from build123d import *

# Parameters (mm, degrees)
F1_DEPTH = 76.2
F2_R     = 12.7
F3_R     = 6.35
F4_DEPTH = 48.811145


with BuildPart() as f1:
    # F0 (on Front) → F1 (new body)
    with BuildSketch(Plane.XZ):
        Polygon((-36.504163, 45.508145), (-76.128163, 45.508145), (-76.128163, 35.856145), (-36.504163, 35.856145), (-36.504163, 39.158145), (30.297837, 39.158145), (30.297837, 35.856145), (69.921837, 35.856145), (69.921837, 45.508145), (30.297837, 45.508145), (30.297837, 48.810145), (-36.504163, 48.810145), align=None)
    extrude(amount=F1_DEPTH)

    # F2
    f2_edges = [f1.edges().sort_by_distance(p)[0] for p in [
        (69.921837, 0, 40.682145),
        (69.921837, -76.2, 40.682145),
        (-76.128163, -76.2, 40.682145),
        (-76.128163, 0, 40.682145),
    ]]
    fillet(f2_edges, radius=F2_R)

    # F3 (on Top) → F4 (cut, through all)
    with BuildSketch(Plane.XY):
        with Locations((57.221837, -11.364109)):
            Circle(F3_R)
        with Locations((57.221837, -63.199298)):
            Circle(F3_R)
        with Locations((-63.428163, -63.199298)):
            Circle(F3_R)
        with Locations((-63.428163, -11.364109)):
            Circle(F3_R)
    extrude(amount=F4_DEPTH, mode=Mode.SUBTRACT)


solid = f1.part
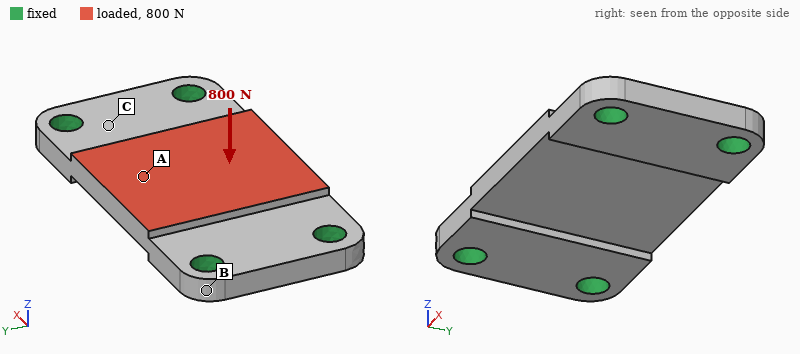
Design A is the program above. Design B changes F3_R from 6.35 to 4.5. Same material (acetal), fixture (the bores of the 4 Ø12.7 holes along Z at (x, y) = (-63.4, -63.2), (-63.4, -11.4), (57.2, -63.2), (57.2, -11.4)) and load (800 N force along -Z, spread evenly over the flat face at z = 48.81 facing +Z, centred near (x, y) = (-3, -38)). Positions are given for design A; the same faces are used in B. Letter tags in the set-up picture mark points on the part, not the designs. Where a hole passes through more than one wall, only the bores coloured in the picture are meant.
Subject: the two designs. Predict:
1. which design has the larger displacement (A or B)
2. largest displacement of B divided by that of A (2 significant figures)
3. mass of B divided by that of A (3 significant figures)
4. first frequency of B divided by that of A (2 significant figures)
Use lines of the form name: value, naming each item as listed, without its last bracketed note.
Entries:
which design has the larger displacement: B
largest displacement of B divided by that of A: 1.2
mass of B divided by that of A: 1.02
first frequency of B divided by that of A: 0.92
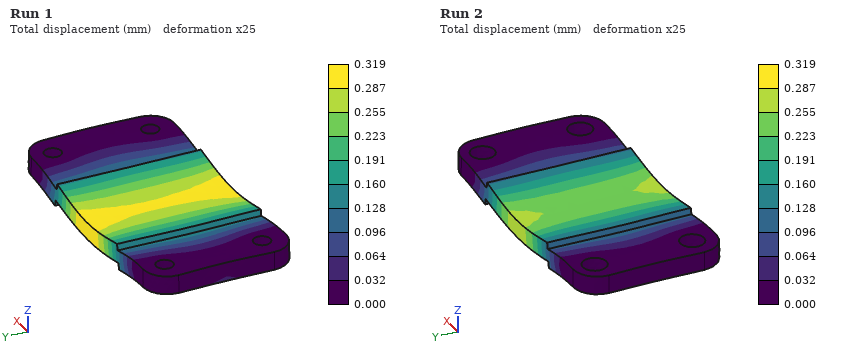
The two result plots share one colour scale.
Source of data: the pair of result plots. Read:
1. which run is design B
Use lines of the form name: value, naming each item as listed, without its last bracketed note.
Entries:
which run is design B: Run 1
